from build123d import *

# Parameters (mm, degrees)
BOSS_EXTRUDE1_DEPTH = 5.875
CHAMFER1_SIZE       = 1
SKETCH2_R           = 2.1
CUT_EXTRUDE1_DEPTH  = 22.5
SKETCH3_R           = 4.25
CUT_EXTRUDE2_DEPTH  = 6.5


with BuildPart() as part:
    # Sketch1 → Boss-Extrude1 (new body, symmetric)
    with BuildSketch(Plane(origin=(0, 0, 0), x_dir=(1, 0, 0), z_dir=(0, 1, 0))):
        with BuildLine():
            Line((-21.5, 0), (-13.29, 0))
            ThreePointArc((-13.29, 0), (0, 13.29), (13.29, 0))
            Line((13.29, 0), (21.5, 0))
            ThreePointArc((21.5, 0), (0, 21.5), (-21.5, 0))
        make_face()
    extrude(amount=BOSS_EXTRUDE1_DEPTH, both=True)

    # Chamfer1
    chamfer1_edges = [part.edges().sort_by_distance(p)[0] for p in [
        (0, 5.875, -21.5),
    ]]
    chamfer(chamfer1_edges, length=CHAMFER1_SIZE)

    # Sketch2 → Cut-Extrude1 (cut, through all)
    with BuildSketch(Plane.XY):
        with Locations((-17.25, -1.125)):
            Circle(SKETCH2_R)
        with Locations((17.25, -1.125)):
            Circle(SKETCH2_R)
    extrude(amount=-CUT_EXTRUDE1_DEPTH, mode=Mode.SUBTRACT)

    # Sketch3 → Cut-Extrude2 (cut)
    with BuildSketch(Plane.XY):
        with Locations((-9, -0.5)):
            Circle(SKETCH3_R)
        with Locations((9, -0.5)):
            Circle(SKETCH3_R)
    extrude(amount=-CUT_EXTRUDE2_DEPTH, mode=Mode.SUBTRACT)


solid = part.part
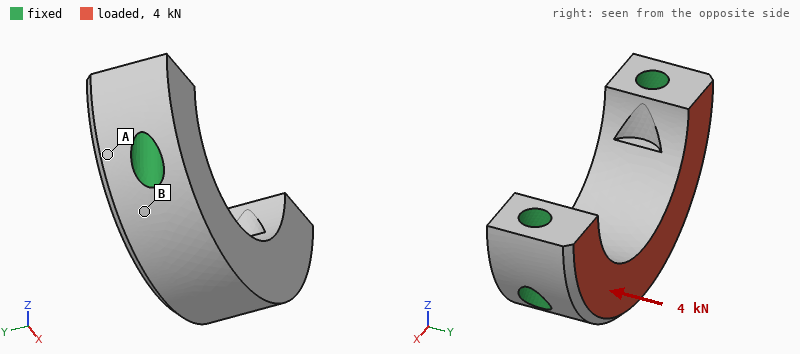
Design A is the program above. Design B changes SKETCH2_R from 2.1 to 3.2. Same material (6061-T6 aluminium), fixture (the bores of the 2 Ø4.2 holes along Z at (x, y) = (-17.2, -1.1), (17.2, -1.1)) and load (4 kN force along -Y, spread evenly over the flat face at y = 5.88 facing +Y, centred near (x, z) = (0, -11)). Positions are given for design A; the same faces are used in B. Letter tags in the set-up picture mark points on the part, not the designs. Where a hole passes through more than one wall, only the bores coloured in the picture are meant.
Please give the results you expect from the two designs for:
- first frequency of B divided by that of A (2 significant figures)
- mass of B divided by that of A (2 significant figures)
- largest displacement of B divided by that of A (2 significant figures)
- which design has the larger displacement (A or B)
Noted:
1.2
0.91
0.67
A
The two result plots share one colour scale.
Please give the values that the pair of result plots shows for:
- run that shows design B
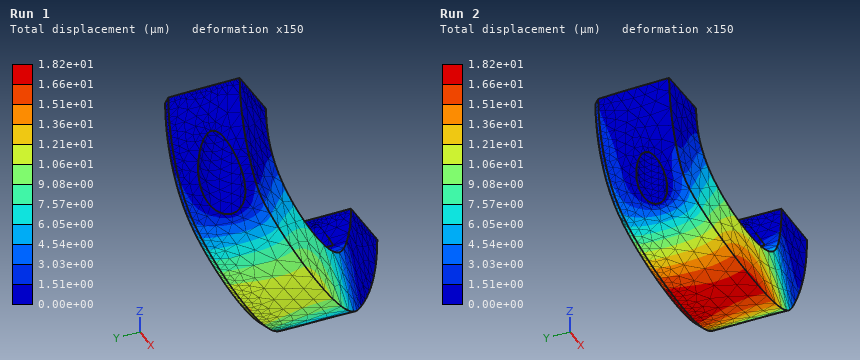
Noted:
Run 1
